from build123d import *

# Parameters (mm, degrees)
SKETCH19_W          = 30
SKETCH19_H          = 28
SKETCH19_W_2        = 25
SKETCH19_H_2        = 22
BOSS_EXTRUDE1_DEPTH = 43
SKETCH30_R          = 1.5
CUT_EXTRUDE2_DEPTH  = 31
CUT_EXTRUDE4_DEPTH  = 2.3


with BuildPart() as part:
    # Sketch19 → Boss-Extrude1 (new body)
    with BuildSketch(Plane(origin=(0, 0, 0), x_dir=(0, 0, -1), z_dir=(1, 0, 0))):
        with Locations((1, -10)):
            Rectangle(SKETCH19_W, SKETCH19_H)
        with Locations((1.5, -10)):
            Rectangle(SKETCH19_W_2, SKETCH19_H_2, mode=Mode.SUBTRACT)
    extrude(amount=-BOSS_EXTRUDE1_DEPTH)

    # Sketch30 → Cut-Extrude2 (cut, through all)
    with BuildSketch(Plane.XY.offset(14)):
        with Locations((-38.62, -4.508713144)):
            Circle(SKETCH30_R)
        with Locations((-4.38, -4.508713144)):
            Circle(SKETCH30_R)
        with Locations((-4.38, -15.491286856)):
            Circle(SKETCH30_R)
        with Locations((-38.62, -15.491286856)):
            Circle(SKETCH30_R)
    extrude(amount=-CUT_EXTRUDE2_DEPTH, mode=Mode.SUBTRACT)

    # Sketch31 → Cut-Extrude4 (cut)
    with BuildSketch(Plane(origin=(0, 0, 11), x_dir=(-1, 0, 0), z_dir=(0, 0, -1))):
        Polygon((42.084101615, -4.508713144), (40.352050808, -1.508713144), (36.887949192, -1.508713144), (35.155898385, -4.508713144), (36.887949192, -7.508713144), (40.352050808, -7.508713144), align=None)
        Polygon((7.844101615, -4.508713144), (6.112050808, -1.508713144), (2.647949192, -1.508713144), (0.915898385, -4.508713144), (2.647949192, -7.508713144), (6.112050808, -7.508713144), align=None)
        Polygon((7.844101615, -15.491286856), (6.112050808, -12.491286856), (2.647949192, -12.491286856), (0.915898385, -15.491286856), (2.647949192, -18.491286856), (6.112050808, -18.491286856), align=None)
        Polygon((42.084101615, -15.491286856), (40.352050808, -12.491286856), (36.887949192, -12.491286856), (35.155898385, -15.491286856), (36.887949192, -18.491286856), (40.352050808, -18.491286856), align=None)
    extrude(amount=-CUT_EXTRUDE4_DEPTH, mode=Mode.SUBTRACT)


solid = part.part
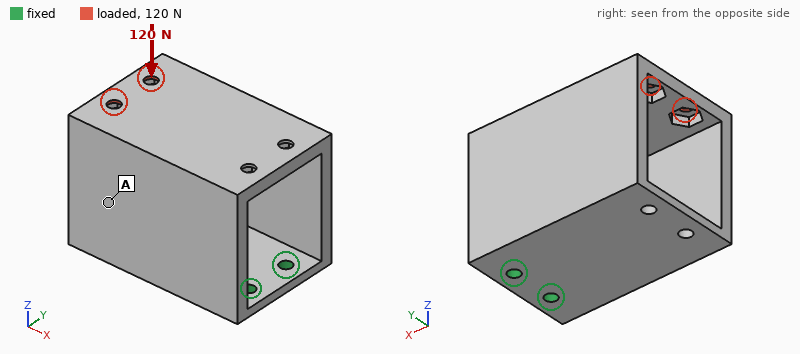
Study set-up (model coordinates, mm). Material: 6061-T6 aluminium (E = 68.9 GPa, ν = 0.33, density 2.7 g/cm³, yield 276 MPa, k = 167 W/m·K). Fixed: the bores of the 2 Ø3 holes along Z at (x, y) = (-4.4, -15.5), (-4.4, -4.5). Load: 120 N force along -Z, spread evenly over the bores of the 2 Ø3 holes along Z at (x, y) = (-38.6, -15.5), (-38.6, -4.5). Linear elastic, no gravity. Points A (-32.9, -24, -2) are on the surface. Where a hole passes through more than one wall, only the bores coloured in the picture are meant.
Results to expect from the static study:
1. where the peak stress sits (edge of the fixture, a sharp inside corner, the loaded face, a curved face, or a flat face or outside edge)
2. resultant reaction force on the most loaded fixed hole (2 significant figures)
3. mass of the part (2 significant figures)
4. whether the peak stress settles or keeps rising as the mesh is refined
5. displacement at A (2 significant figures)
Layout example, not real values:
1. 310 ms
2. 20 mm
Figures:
1. edge of the fixture
2. 64 N
3. 33 g
4. keeps rising
5. 0.26 mm
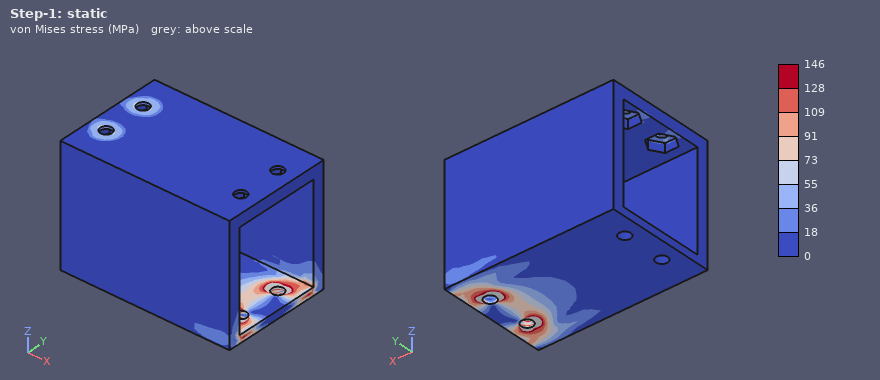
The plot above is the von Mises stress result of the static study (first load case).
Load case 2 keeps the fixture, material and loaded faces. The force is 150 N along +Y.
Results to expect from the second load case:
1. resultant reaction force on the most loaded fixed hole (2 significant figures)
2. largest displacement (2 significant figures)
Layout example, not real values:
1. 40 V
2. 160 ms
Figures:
1. 440 N
2. 0.15 mm
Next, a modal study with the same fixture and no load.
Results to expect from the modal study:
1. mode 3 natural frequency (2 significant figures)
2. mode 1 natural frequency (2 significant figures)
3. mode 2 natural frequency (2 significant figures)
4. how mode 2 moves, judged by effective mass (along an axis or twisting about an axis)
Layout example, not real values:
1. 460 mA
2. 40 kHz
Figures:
1. 3300 Hz
2. 700 Hz
3. 1200 Hz
4. along Y
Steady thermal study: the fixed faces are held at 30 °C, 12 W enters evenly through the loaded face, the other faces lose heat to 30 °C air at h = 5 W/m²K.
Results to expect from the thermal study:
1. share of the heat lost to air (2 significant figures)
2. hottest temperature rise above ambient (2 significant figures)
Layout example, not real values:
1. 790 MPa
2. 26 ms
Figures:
1. 6.1 %
2. 36 K
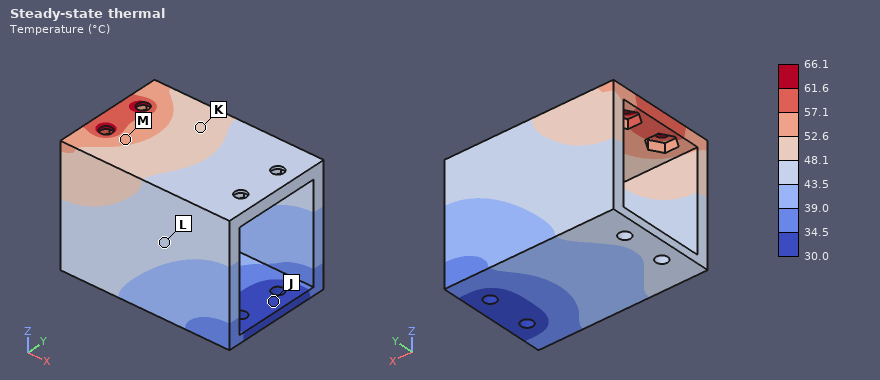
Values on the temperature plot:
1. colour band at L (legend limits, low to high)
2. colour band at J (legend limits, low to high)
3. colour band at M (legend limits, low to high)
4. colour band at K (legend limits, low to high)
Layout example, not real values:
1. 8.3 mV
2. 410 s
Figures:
1. 43.5 to 48.1 °C
2. 30.0 to 34.5 °C
3. 52.6 to 57.1 °C
4. 48.1 to 52.6 °C
